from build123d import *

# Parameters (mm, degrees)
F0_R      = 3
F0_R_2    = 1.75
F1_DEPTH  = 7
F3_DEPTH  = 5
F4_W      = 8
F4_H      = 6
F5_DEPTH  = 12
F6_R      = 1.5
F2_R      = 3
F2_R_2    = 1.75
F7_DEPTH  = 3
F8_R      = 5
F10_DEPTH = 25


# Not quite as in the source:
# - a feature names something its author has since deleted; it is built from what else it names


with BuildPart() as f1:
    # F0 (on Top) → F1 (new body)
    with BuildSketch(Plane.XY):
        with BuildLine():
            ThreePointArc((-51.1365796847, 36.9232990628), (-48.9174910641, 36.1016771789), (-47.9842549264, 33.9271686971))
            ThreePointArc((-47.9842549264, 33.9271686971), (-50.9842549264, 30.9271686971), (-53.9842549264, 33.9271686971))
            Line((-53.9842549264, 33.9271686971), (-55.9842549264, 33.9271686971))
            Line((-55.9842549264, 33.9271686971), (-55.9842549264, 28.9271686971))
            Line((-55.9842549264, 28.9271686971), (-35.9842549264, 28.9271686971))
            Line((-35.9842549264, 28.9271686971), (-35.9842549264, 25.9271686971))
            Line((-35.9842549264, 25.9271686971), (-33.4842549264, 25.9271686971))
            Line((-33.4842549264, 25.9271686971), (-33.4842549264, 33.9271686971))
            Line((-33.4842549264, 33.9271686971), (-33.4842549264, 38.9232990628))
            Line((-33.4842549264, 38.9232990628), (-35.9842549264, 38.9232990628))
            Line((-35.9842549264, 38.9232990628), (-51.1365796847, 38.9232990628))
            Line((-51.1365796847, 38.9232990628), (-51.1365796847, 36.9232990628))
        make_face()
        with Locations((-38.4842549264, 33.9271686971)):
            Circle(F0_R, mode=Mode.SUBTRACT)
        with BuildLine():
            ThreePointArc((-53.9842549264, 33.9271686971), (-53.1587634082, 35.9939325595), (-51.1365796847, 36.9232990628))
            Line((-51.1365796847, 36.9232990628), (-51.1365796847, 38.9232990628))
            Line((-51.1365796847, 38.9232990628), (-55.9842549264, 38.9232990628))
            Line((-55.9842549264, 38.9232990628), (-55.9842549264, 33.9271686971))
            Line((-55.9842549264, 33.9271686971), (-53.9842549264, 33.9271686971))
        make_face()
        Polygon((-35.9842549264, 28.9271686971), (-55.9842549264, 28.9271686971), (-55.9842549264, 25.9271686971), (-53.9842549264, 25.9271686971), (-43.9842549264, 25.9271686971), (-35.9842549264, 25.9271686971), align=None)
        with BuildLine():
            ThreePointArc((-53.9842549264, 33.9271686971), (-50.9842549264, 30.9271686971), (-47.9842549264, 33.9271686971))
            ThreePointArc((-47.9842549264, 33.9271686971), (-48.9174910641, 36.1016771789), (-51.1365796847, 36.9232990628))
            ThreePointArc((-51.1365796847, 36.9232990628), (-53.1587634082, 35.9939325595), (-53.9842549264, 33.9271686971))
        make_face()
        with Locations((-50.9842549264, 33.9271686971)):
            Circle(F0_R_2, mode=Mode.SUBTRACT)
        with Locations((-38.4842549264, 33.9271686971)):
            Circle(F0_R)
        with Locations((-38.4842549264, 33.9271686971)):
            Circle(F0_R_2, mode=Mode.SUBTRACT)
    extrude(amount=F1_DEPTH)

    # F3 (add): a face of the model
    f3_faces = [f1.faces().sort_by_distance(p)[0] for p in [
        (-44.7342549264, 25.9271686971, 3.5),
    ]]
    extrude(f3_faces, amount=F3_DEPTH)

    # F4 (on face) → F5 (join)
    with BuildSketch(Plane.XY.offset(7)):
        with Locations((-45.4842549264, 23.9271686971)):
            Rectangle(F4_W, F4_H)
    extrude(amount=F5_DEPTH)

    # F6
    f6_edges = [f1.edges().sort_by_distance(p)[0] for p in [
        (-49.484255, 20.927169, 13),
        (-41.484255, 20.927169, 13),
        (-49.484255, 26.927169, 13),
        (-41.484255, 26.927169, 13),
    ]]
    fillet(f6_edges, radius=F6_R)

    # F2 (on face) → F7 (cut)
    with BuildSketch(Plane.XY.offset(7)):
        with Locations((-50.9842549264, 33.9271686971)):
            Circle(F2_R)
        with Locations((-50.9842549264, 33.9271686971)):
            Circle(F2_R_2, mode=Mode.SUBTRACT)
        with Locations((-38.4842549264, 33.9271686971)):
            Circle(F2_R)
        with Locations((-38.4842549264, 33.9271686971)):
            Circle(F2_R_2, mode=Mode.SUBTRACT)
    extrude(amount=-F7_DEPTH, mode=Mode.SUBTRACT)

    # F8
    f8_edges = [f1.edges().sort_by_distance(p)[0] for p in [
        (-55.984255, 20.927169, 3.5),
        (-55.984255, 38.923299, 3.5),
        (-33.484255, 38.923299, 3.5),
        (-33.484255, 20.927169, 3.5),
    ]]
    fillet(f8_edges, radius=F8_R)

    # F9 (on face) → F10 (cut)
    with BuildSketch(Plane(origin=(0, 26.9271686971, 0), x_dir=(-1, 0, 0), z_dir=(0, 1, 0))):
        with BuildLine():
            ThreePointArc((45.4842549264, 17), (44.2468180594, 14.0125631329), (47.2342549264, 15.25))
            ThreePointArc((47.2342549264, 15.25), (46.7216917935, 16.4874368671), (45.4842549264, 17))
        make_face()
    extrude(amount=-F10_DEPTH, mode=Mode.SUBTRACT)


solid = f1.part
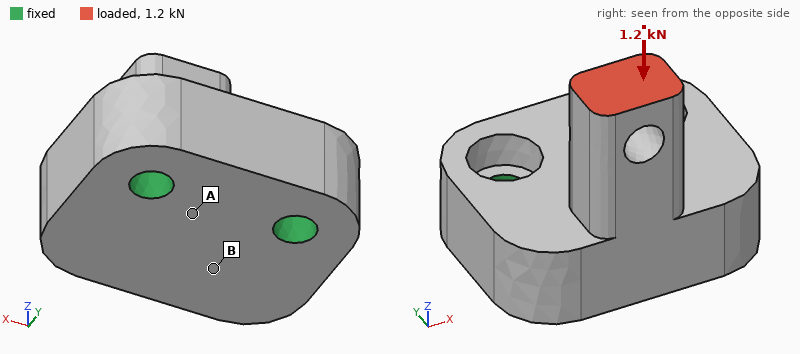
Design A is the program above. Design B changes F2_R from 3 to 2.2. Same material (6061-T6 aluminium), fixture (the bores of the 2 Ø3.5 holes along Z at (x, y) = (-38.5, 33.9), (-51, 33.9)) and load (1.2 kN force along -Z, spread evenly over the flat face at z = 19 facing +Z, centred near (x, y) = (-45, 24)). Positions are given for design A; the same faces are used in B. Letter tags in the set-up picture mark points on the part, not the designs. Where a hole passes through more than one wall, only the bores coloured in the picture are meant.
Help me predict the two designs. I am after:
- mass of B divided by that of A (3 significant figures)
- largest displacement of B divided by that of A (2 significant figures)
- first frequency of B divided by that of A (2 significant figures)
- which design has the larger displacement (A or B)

1.03
0.91
1.0
A
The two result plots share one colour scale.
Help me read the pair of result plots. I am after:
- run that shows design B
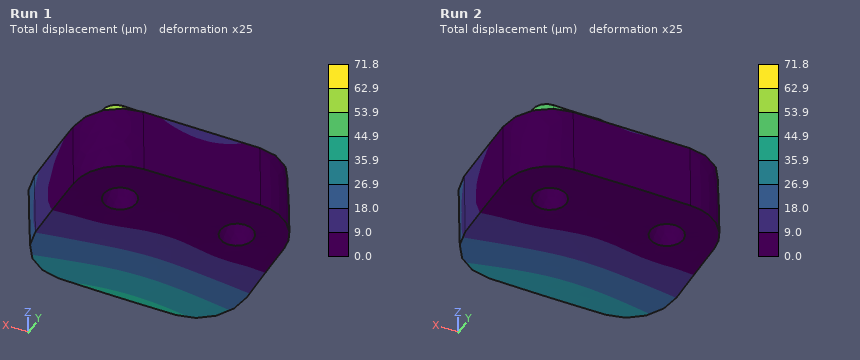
Run 2
